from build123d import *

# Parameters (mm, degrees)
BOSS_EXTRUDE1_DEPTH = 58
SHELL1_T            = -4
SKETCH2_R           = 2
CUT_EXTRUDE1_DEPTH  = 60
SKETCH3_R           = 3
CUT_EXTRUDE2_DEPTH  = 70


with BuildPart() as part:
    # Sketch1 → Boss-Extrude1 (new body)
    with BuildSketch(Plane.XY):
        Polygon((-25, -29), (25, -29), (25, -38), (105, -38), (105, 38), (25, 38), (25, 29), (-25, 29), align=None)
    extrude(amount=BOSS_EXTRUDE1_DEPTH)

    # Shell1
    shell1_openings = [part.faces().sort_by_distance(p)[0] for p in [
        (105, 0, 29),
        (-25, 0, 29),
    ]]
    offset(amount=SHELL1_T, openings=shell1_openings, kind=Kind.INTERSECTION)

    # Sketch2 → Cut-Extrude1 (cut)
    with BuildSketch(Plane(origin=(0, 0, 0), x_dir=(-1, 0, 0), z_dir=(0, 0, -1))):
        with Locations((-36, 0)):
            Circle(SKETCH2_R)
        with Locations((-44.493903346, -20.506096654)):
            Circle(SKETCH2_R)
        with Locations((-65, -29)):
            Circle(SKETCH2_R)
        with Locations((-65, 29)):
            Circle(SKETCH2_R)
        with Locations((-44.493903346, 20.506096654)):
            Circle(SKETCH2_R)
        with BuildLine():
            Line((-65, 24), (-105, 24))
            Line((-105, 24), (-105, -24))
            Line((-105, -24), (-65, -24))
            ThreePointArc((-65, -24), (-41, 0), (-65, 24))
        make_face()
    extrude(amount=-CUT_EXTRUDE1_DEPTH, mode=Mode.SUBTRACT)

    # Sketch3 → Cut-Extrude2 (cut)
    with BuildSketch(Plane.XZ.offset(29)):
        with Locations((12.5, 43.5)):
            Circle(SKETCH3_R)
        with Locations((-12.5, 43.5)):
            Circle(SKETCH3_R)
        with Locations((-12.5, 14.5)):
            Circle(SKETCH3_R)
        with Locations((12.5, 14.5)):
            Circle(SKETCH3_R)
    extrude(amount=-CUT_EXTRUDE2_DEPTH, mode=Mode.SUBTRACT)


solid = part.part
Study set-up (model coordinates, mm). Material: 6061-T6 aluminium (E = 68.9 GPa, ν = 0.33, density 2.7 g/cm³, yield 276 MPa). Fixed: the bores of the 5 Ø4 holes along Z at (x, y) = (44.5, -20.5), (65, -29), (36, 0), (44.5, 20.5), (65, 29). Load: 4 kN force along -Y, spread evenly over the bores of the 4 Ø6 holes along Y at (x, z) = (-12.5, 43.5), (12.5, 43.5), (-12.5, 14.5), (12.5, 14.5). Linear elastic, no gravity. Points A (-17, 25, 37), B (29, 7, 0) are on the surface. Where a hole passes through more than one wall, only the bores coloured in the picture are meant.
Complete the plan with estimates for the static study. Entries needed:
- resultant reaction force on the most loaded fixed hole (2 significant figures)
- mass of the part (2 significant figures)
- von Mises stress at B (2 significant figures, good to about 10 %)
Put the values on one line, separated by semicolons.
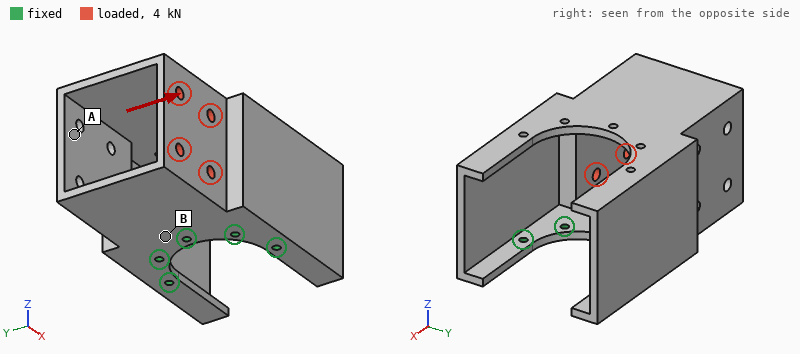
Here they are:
2.2 kN; 280 g; 44 MPa
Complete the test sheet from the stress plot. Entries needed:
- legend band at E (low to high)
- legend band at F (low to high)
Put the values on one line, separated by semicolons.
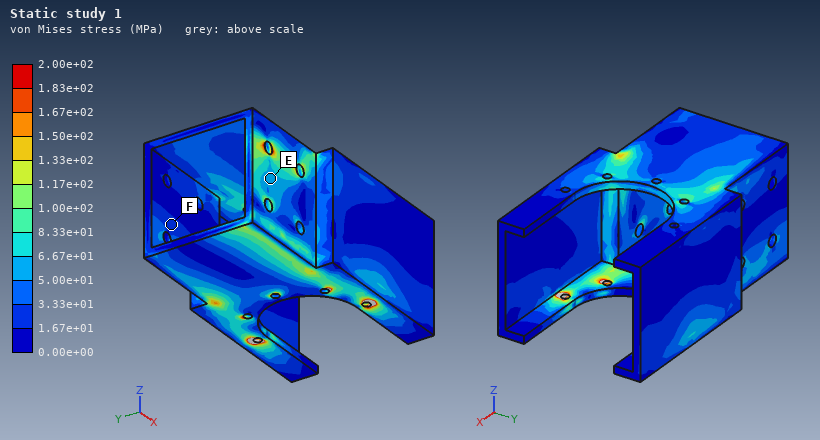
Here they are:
5.00e+01 to 6.67e+01 MPa; 1.67e+01 to 3.33e+01 MPa
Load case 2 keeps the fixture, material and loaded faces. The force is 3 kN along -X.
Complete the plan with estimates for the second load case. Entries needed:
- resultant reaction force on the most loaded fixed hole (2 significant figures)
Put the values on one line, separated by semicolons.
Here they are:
2.1 kN
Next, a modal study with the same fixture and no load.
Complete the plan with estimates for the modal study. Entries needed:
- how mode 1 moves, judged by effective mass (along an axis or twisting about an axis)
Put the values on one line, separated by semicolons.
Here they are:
along Y
